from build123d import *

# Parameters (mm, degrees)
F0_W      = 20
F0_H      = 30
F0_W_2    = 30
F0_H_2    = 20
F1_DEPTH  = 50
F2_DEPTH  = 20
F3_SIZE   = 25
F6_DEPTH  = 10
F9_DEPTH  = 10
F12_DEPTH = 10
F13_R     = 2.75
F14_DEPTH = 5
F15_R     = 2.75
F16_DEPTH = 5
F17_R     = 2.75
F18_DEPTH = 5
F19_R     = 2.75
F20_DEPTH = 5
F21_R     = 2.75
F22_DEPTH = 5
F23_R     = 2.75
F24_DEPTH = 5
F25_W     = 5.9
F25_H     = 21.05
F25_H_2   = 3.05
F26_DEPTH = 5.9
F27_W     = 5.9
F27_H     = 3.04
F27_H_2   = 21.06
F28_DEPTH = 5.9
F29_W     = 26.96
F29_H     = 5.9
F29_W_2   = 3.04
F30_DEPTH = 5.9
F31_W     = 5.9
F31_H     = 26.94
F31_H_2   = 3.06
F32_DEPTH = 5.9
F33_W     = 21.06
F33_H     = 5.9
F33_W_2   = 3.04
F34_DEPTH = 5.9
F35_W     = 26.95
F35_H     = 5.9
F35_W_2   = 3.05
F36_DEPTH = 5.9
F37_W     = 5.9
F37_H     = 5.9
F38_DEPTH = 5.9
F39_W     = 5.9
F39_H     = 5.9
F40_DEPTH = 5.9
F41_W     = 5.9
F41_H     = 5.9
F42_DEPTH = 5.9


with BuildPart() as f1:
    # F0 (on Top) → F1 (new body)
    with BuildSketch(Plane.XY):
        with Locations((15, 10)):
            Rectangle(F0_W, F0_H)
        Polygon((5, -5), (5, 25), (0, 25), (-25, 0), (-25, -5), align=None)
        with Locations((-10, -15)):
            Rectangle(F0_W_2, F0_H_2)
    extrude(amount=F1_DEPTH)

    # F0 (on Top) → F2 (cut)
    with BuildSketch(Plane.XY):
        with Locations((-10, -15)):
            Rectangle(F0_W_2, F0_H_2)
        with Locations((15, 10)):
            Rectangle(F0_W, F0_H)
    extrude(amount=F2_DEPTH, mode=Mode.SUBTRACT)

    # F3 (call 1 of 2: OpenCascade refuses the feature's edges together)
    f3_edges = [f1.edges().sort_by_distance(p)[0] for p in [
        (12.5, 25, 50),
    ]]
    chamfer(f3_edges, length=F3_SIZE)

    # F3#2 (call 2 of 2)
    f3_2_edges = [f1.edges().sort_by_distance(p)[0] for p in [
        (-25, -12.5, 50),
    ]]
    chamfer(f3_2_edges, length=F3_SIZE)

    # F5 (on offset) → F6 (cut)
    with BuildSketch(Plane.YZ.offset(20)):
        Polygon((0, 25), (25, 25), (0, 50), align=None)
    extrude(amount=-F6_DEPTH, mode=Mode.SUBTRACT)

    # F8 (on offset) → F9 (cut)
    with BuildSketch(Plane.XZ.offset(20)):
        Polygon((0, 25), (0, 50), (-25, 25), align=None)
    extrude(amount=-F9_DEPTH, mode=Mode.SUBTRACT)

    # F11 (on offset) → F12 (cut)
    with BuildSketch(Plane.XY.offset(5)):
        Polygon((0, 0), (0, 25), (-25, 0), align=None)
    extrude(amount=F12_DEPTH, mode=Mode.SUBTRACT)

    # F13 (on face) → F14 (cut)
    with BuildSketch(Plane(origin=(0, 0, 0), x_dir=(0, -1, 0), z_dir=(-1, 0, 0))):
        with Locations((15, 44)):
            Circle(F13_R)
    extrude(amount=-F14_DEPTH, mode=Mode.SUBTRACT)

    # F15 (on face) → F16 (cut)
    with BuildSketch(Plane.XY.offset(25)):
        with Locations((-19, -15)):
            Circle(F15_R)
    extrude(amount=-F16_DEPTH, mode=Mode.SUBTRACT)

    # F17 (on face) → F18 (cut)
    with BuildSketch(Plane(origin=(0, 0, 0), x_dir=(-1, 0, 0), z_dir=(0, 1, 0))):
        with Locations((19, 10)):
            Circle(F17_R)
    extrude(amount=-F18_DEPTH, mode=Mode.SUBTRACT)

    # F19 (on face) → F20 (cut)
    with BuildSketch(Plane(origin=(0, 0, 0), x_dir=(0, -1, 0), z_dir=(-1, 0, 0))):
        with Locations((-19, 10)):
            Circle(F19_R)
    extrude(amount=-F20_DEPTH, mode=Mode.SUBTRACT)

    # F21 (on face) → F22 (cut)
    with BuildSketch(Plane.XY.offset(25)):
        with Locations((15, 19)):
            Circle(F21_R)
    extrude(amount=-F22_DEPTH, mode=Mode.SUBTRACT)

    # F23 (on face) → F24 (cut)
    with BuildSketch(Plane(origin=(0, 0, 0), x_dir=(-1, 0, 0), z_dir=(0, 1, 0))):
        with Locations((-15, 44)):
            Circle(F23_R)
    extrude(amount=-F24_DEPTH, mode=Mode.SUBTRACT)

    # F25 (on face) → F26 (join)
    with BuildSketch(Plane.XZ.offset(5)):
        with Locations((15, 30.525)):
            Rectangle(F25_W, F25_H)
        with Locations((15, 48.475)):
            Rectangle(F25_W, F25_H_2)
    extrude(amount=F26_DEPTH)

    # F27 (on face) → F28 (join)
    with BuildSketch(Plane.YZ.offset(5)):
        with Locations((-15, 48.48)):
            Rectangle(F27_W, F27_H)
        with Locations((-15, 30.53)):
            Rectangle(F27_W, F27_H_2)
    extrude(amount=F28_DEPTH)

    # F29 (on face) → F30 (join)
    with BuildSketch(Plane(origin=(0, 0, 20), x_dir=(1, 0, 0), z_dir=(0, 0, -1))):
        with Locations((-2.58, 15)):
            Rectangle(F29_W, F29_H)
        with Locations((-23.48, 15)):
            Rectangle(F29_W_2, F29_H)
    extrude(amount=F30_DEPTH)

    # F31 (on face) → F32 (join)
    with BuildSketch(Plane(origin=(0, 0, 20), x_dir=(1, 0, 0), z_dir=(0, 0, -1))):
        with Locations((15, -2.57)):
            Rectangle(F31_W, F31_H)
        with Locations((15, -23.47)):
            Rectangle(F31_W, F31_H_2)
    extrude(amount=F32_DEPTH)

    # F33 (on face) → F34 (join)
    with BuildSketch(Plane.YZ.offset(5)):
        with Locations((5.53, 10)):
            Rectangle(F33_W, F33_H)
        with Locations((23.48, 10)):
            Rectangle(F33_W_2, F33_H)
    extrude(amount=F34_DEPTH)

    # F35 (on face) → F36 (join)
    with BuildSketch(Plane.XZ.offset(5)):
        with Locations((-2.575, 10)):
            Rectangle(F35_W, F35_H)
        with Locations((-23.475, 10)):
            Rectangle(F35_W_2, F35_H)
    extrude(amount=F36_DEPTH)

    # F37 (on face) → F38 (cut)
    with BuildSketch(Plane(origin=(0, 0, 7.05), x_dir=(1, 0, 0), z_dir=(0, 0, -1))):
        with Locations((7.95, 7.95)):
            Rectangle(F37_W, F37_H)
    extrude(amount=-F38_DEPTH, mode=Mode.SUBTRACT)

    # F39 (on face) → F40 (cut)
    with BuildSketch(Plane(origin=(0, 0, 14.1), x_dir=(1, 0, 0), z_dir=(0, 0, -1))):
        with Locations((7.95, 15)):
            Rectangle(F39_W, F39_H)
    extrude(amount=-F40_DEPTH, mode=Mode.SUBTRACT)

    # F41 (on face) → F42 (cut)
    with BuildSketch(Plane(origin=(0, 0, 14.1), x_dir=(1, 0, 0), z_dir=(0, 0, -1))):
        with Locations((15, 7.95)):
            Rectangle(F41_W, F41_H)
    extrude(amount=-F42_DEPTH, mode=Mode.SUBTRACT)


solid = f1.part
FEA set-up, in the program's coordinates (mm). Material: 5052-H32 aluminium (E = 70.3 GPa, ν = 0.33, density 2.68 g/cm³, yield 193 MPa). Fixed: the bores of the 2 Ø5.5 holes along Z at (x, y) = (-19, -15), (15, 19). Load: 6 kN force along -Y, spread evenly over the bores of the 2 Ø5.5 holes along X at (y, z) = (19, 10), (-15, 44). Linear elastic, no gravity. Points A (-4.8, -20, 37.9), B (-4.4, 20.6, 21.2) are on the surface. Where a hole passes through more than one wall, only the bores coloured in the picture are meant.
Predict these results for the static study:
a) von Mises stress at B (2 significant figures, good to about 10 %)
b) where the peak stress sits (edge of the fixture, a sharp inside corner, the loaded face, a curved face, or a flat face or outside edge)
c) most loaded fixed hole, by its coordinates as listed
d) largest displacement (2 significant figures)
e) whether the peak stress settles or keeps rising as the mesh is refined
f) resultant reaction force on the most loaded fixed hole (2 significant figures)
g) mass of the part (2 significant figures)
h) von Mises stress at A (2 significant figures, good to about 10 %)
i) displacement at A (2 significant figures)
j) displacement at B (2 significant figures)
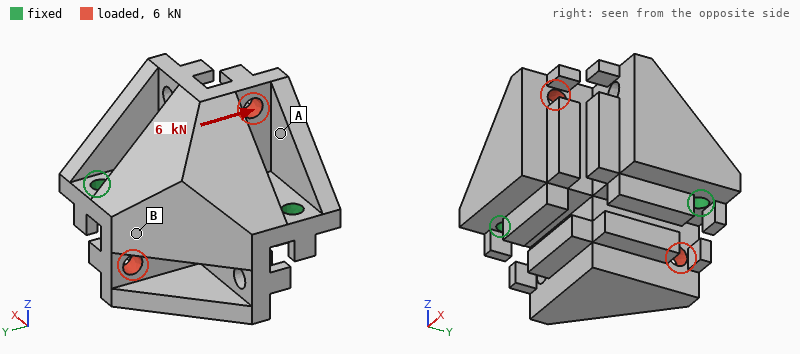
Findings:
36 MPa
edge of the fixture
(15, 19)
84 µm
keeps rising
3.3 kN
110 g
12 MPa
47 µm
23 µm
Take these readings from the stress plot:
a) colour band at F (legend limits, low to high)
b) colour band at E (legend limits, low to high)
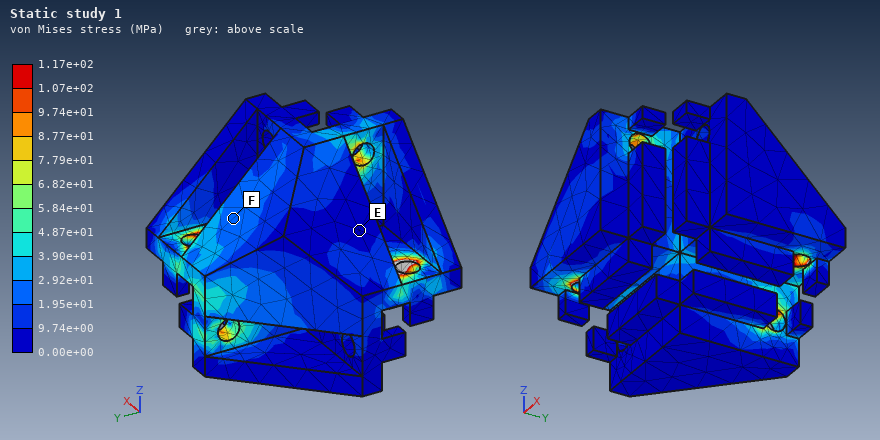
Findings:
1.95e+01 to 2.92e+01 MPa
0.00e+00 to 9.74e+00 MPa
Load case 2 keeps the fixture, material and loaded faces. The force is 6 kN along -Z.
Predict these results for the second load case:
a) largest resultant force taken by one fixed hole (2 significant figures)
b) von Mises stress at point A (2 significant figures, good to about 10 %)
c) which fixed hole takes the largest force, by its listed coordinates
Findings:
3.6 kN
27 MPa
(15, 19)
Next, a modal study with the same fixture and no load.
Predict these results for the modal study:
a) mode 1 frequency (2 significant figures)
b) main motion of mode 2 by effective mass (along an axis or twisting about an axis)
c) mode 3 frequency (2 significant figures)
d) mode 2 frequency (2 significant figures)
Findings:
3300 Hz
along Z
10 kHz
9100 Hz
